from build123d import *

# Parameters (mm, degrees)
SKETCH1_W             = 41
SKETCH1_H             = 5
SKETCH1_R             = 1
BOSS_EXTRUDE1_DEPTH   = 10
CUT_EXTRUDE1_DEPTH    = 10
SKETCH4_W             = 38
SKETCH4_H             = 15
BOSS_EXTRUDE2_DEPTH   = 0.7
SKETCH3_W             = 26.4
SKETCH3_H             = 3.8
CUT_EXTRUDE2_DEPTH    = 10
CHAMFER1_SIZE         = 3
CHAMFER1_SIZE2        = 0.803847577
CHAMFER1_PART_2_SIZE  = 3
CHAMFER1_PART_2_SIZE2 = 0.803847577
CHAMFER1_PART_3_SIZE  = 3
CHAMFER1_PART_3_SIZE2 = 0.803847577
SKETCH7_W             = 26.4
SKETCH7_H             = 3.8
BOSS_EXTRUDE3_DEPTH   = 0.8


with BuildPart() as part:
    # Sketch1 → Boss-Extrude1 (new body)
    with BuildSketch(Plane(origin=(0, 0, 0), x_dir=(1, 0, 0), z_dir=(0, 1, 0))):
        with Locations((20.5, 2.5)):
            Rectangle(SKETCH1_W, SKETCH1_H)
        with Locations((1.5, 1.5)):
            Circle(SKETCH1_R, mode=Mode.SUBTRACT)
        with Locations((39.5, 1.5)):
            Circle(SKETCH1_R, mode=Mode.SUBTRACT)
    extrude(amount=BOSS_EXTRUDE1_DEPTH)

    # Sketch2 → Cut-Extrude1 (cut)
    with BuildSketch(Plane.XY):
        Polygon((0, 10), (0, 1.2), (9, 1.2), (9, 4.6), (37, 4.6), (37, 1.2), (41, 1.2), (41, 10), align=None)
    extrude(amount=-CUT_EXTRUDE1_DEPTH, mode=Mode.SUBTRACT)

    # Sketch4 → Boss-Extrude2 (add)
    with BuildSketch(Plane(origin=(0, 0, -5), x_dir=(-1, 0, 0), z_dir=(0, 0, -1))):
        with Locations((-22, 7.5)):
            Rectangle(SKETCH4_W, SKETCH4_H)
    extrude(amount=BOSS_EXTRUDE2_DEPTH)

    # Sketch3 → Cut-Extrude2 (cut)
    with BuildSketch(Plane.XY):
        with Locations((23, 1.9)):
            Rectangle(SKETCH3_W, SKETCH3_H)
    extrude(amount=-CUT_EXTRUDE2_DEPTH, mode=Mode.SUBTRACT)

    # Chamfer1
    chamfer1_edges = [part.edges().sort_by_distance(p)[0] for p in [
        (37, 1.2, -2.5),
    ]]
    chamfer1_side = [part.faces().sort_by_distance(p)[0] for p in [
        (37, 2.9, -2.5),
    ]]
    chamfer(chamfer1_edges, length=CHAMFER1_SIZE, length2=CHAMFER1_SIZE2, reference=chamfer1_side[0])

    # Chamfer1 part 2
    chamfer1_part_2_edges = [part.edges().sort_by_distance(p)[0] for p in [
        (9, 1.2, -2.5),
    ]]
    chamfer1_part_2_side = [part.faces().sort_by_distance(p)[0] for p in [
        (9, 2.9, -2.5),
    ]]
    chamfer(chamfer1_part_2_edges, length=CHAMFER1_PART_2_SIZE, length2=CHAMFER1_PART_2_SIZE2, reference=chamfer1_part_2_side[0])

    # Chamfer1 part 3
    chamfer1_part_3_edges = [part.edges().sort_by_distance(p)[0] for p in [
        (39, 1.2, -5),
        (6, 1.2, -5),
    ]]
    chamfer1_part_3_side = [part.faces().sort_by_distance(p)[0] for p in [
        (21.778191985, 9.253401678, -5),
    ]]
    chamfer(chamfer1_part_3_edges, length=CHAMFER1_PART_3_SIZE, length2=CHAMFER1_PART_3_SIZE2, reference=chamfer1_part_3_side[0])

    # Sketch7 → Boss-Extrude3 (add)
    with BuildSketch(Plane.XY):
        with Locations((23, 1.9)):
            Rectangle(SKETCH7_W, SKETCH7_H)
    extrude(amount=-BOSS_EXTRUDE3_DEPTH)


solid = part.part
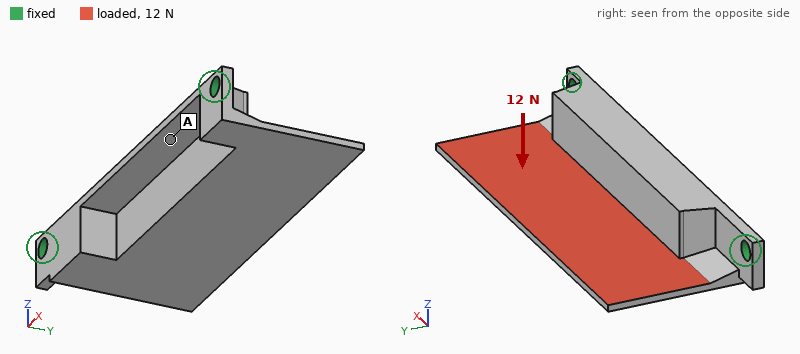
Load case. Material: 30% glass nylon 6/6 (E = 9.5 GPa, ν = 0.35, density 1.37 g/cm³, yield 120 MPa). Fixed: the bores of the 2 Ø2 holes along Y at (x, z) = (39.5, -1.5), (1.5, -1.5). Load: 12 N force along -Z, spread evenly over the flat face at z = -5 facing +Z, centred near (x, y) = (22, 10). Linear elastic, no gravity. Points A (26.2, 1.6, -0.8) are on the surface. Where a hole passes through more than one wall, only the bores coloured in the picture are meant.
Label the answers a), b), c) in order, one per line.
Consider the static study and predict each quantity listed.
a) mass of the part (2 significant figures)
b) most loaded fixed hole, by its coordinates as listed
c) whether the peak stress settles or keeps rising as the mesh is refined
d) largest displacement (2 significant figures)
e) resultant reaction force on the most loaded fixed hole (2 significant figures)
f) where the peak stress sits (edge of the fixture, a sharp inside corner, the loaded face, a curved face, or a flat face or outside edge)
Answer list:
a) 0.88 g
b) (39.5, -1.5)
c) keeps rising
d) 0.45 mm
e) 9.0 N
f) edge of the fixture
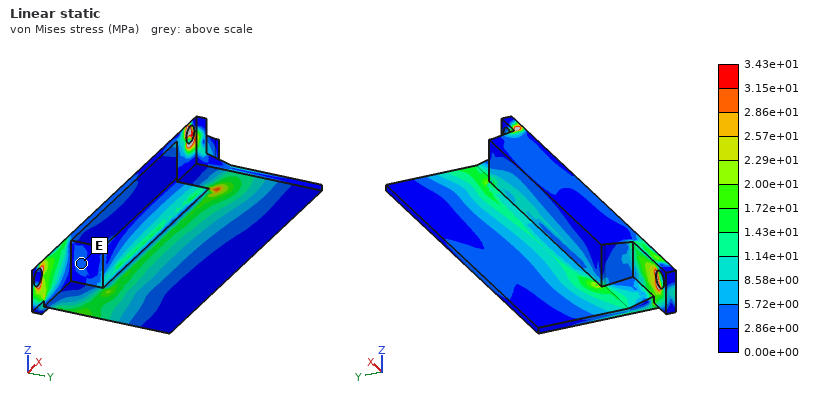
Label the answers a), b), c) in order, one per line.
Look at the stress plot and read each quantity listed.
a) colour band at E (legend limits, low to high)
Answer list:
a) 2.86e+00 to 5.72e+00 MPa
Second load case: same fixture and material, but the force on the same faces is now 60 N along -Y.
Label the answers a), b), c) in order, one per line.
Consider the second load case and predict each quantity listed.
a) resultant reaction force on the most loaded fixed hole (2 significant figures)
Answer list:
a) 37 N
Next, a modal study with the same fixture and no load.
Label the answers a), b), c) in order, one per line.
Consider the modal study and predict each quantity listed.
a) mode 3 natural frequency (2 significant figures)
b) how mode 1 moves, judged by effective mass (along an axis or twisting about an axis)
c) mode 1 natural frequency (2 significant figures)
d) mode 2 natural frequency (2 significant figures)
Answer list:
a) 3900 Hz
b) along Z
c) 1700 Hz
d) 2600 Hz
